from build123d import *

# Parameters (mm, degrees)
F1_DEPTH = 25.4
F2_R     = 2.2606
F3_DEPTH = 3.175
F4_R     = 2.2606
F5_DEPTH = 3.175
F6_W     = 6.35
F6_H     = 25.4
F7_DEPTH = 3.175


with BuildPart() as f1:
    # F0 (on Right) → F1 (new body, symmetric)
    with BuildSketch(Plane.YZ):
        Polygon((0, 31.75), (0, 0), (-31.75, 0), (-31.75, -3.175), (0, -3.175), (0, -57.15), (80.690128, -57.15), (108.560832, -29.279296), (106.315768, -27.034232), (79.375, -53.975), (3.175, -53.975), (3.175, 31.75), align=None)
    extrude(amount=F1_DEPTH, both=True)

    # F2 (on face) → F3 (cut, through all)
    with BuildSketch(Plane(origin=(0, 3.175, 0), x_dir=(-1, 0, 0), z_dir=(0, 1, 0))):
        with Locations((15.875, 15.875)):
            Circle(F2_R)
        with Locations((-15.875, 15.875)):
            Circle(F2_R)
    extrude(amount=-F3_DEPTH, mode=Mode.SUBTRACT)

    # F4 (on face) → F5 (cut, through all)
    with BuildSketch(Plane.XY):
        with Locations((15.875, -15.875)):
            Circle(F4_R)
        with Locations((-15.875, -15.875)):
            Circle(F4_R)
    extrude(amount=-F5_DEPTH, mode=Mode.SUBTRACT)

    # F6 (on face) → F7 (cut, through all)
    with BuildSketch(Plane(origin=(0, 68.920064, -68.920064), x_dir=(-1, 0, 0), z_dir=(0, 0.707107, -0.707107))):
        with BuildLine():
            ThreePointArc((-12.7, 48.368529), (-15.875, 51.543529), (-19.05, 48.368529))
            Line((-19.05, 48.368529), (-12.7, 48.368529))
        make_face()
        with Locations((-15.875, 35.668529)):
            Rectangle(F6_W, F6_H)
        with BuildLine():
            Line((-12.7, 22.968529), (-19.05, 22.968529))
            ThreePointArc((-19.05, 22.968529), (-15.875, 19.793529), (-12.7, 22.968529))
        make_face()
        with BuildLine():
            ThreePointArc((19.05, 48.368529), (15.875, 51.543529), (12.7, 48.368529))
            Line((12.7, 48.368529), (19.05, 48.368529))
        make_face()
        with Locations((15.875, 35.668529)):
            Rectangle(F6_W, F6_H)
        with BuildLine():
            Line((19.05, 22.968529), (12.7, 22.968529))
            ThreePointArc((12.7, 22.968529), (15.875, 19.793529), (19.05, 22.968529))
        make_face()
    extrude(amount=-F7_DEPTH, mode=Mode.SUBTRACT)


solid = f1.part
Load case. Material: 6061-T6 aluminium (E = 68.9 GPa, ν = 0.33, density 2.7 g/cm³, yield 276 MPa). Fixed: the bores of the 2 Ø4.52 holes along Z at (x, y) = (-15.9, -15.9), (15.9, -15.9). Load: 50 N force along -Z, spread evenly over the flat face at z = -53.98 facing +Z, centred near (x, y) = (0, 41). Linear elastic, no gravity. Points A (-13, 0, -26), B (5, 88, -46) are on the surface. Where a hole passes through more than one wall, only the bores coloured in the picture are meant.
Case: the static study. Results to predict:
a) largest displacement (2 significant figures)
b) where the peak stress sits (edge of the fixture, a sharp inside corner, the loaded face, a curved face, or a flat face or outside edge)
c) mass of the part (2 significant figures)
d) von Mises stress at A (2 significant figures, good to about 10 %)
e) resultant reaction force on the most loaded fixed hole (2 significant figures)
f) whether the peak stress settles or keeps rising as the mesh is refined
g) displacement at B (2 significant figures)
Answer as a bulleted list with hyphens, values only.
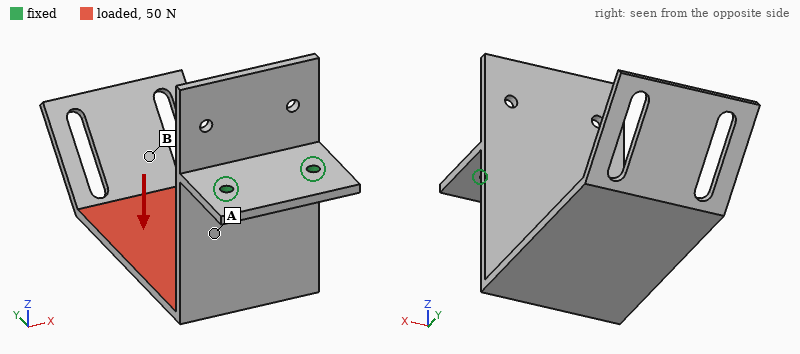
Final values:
- 2.0 mm
- edge of the fixture
- 99 g
- 21 MPa
- 27 N
- keeps rising
- 1.6 mm
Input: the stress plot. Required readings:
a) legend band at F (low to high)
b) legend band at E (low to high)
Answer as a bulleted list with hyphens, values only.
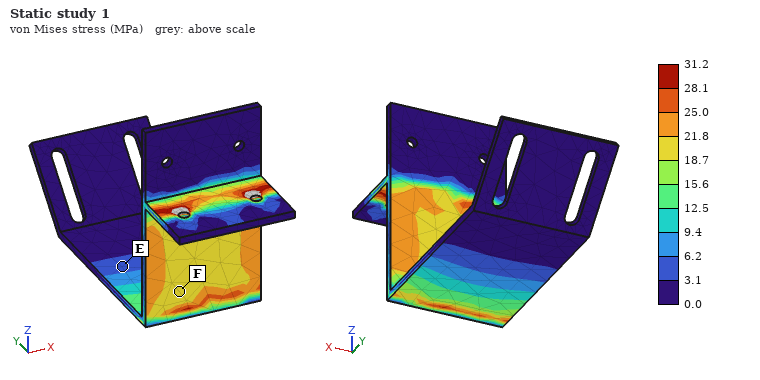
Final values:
- 18.7 to 21.8 MPa
- 3.1 to 6.2 MPa
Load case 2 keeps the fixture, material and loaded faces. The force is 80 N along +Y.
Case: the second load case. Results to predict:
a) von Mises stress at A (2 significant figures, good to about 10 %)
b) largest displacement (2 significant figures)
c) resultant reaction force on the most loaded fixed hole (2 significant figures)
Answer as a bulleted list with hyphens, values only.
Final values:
- 24 MPa
- 1.9 mm
- 45 N
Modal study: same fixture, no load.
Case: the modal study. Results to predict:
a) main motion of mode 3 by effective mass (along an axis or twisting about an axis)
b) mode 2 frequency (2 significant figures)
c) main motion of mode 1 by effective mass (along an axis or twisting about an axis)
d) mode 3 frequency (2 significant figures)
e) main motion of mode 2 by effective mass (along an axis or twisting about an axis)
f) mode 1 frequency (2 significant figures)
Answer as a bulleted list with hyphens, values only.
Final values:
- along Y
- 210 Hz
- along Z
- 340 Hz
- along X
- 110 Hz
